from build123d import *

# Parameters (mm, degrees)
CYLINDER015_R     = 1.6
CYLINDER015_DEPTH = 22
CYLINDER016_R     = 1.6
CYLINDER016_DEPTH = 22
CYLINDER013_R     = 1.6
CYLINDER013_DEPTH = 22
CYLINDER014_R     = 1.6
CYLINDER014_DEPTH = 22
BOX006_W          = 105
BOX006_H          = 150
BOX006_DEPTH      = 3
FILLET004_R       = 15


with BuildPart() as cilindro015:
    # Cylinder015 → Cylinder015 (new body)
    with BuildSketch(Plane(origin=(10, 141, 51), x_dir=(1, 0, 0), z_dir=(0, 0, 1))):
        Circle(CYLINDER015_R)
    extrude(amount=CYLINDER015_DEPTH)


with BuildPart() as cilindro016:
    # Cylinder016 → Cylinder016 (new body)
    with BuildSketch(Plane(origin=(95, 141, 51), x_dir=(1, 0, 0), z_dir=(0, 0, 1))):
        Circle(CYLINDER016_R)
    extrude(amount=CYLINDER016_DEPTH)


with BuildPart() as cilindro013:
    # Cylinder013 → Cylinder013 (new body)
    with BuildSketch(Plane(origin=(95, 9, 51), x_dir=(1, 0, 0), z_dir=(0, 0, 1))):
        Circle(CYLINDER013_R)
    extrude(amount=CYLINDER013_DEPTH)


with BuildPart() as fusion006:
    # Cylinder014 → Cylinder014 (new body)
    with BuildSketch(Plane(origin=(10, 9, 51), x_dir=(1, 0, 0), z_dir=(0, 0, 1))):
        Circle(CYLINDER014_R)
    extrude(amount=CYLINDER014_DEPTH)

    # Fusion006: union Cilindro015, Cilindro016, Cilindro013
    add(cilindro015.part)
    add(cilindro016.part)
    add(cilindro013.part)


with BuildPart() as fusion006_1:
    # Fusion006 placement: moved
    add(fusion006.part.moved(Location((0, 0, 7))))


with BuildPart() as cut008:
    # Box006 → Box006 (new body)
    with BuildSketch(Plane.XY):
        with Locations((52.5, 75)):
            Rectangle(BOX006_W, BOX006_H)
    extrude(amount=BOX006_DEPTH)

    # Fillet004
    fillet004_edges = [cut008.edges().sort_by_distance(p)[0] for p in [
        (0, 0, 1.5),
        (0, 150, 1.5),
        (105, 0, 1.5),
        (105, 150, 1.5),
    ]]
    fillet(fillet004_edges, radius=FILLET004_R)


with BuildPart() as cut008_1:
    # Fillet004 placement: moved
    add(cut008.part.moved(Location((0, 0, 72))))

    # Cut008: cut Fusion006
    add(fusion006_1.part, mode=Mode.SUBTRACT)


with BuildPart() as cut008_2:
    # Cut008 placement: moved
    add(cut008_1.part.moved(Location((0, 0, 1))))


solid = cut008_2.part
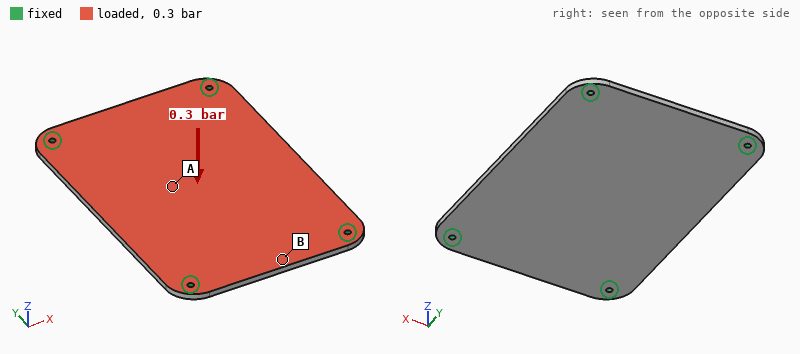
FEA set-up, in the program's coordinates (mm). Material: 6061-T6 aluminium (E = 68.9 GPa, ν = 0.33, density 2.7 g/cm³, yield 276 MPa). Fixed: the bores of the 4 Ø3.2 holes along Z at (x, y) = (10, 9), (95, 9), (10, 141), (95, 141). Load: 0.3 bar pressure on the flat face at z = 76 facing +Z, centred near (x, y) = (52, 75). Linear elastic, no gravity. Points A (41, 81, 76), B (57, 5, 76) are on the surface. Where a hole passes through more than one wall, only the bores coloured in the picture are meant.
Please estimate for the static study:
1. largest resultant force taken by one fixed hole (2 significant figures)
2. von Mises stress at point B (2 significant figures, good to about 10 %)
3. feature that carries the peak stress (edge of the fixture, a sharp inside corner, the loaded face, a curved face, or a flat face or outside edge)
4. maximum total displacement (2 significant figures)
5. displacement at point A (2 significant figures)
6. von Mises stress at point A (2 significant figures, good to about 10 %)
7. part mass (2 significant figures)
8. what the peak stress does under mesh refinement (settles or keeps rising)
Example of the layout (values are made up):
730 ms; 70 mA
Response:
120 N; 8.2 MPa; edge of the fixture; 0.25 mm; 0.24 mm; 16 MPa; 130 g; keeps rising
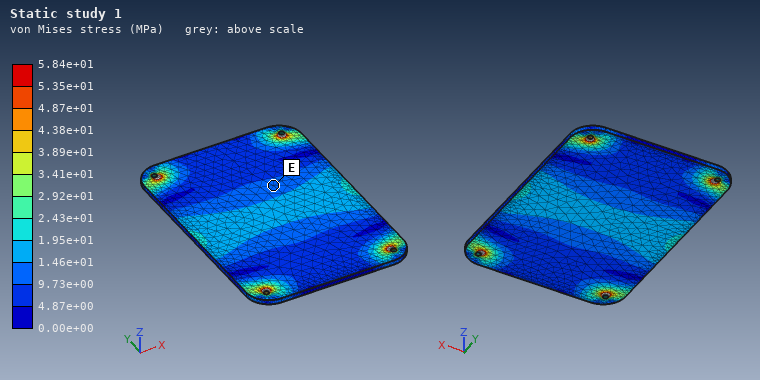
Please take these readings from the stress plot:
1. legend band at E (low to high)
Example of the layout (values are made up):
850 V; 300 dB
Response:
9.73e+00 to 1.46e+01 MPa
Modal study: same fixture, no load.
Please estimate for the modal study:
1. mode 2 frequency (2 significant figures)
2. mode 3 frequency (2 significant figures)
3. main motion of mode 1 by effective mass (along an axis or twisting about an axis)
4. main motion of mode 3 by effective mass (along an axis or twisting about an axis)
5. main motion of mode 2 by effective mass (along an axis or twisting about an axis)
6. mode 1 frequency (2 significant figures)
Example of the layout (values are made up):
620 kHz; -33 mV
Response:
1100 Hz; 1800 Hz; along Z; twisting about X; twisting about Y; 710 Hz
